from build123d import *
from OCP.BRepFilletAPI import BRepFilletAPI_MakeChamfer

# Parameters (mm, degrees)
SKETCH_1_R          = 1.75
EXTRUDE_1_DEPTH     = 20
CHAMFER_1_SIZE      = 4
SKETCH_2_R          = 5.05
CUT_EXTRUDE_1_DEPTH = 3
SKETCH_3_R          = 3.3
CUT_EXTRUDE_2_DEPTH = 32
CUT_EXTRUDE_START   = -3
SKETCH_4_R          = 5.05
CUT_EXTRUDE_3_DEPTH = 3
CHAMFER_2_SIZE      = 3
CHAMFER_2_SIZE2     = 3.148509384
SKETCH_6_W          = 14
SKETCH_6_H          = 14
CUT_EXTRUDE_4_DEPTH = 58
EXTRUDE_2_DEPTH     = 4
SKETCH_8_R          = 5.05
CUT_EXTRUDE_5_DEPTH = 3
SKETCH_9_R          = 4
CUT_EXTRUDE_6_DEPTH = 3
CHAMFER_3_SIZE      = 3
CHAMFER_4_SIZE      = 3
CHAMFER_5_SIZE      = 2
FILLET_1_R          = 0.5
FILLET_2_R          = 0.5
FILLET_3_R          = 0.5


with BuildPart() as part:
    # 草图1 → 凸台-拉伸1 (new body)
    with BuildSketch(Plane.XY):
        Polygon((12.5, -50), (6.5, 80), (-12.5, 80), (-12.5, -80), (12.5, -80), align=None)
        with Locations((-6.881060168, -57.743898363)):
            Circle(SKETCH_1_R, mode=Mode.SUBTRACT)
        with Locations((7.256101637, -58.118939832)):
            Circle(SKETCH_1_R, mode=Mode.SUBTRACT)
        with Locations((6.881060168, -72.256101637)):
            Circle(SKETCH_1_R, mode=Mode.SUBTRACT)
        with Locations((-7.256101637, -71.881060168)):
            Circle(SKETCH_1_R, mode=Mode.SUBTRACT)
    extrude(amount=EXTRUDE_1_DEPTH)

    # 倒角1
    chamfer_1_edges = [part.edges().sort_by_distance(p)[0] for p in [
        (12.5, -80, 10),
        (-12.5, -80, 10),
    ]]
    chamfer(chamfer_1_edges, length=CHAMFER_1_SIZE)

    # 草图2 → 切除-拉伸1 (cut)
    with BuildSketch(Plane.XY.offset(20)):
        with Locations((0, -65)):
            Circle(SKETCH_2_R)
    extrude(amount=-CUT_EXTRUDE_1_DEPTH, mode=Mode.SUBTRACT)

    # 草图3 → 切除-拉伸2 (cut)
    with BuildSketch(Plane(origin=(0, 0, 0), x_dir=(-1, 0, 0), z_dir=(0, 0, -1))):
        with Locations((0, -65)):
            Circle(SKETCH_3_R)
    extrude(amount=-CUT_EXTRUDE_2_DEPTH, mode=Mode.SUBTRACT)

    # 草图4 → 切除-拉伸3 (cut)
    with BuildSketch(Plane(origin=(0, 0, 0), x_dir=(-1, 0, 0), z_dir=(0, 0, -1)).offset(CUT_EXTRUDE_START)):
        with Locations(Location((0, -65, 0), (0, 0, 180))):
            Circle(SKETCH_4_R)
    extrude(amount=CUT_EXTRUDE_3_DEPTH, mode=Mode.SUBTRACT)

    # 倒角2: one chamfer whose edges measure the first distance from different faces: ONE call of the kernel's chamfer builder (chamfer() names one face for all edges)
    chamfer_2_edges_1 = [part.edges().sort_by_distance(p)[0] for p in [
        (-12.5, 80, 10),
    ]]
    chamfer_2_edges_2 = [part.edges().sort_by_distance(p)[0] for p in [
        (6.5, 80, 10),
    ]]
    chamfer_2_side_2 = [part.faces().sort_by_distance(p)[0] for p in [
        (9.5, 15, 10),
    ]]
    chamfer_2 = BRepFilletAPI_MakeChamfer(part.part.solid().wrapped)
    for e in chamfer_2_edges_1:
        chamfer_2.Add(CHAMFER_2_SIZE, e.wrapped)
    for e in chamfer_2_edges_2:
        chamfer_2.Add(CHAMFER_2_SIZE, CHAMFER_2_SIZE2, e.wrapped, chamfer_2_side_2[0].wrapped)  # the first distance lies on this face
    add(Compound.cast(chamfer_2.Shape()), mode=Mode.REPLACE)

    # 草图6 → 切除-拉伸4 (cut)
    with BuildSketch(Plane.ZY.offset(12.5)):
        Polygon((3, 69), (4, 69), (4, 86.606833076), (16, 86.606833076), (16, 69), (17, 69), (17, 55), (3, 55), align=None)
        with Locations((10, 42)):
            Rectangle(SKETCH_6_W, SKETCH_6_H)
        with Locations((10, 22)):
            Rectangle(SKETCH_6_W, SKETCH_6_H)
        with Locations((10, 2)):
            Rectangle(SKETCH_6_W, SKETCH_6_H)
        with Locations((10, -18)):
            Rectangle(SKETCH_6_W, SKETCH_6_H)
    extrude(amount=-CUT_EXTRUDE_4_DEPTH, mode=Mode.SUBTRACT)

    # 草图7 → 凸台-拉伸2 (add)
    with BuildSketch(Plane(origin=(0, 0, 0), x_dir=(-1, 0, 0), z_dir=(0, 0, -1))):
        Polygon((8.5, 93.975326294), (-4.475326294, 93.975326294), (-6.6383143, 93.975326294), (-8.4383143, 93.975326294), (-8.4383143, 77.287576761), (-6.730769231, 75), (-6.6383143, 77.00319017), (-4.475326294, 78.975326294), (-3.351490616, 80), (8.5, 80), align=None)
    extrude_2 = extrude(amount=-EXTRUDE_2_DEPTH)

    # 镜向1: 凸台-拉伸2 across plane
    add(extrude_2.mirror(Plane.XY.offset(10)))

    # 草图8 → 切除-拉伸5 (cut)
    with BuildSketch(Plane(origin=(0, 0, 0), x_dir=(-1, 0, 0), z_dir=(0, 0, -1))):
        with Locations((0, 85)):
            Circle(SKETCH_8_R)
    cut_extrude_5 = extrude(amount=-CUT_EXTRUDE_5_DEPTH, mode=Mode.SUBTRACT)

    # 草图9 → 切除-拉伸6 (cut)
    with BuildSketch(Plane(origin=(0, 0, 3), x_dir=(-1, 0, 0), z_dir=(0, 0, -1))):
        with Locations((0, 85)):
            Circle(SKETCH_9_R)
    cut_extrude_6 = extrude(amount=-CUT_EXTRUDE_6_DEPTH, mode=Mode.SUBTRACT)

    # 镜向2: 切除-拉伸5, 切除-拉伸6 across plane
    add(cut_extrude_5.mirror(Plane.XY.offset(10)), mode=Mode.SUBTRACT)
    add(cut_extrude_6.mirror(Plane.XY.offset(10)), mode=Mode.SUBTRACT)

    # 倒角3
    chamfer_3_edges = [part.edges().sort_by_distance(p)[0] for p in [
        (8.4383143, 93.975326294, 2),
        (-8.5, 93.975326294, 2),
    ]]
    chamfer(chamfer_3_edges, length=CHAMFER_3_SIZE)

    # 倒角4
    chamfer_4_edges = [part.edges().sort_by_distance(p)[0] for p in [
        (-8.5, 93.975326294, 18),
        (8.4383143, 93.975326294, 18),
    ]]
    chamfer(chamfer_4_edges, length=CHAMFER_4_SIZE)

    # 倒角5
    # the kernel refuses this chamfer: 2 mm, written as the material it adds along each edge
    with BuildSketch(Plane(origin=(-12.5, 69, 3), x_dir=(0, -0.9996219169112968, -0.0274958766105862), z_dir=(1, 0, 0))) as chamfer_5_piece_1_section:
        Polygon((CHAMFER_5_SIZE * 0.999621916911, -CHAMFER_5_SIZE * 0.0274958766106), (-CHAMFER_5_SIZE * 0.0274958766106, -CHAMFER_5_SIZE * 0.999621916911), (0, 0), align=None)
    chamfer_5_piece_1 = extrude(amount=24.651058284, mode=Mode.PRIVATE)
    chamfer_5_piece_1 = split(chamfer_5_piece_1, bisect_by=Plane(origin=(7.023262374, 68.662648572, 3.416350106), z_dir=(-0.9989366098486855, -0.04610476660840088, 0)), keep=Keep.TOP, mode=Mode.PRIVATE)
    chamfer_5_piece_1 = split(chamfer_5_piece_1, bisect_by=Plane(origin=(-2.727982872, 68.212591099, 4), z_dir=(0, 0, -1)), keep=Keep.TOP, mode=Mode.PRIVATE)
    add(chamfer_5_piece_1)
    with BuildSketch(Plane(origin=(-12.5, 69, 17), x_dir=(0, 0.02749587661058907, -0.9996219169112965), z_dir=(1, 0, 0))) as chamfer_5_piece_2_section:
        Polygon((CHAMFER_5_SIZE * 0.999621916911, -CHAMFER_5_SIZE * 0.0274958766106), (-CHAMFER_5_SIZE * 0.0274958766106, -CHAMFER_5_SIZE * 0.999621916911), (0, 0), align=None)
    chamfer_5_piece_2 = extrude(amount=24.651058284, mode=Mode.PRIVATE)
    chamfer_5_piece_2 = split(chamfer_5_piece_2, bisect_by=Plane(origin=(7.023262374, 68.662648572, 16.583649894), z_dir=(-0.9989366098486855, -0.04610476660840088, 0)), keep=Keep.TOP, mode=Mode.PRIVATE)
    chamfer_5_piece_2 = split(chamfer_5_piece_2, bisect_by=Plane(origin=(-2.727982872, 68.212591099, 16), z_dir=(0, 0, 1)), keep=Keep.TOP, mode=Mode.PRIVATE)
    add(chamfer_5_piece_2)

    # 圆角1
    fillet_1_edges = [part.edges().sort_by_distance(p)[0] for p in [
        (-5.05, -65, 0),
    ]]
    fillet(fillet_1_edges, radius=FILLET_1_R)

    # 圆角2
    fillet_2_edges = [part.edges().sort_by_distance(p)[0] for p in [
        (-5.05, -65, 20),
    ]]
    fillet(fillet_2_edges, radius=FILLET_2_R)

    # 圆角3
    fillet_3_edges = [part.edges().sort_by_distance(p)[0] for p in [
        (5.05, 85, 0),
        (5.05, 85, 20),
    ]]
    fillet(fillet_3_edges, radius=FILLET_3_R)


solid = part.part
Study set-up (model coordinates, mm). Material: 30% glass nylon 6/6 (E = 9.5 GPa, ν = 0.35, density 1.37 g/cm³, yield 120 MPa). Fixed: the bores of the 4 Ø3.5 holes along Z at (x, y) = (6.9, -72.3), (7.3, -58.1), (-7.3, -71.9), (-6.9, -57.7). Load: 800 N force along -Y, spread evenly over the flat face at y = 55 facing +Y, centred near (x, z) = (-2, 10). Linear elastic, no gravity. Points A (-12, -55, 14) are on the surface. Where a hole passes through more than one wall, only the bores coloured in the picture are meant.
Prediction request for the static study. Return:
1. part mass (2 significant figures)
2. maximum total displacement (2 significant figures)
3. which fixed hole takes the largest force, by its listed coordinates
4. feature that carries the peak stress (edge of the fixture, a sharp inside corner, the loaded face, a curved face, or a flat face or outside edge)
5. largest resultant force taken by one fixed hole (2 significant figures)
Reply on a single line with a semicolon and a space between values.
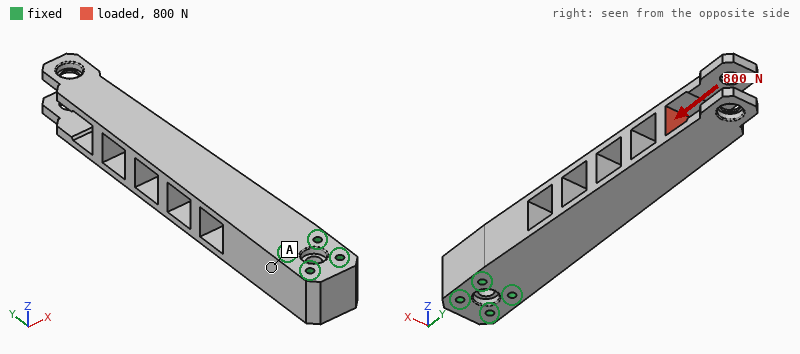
65 g; 0.18 mm; (-6.9, -57.7); a flat face or outside edge; 480 N
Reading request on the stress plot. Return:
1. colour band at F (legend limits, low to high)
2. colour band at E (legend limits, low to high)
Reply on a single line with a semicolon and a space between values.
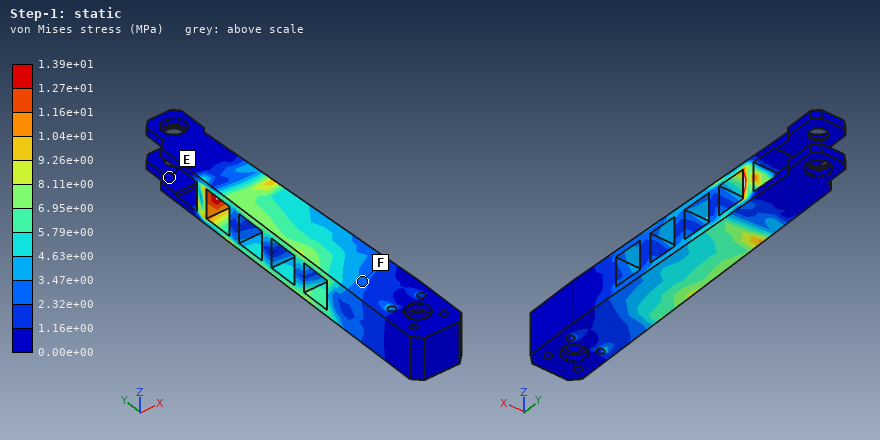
2.32e+00 to 3.47e+00 MPa; 0.00e+00 to 1.16e+00 MPa
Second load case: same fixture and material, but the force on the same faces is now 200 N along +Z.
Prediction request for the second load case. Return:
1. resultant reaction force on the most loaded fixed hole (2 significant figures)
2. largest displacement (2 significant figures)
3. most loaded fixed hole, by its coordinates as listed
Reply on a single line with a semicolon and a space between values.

180 N; 1.4 mm; (-6.9, -57.7)
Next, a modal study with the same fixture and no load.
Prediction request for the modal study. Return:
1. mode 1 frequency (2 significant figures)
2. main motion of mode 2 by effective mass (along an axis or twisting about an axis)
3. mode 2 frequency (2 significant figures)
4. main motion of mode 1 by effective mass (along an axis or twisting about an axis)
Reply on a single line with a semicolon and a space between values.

490 Hz; along X; 540 Hz; along Z
